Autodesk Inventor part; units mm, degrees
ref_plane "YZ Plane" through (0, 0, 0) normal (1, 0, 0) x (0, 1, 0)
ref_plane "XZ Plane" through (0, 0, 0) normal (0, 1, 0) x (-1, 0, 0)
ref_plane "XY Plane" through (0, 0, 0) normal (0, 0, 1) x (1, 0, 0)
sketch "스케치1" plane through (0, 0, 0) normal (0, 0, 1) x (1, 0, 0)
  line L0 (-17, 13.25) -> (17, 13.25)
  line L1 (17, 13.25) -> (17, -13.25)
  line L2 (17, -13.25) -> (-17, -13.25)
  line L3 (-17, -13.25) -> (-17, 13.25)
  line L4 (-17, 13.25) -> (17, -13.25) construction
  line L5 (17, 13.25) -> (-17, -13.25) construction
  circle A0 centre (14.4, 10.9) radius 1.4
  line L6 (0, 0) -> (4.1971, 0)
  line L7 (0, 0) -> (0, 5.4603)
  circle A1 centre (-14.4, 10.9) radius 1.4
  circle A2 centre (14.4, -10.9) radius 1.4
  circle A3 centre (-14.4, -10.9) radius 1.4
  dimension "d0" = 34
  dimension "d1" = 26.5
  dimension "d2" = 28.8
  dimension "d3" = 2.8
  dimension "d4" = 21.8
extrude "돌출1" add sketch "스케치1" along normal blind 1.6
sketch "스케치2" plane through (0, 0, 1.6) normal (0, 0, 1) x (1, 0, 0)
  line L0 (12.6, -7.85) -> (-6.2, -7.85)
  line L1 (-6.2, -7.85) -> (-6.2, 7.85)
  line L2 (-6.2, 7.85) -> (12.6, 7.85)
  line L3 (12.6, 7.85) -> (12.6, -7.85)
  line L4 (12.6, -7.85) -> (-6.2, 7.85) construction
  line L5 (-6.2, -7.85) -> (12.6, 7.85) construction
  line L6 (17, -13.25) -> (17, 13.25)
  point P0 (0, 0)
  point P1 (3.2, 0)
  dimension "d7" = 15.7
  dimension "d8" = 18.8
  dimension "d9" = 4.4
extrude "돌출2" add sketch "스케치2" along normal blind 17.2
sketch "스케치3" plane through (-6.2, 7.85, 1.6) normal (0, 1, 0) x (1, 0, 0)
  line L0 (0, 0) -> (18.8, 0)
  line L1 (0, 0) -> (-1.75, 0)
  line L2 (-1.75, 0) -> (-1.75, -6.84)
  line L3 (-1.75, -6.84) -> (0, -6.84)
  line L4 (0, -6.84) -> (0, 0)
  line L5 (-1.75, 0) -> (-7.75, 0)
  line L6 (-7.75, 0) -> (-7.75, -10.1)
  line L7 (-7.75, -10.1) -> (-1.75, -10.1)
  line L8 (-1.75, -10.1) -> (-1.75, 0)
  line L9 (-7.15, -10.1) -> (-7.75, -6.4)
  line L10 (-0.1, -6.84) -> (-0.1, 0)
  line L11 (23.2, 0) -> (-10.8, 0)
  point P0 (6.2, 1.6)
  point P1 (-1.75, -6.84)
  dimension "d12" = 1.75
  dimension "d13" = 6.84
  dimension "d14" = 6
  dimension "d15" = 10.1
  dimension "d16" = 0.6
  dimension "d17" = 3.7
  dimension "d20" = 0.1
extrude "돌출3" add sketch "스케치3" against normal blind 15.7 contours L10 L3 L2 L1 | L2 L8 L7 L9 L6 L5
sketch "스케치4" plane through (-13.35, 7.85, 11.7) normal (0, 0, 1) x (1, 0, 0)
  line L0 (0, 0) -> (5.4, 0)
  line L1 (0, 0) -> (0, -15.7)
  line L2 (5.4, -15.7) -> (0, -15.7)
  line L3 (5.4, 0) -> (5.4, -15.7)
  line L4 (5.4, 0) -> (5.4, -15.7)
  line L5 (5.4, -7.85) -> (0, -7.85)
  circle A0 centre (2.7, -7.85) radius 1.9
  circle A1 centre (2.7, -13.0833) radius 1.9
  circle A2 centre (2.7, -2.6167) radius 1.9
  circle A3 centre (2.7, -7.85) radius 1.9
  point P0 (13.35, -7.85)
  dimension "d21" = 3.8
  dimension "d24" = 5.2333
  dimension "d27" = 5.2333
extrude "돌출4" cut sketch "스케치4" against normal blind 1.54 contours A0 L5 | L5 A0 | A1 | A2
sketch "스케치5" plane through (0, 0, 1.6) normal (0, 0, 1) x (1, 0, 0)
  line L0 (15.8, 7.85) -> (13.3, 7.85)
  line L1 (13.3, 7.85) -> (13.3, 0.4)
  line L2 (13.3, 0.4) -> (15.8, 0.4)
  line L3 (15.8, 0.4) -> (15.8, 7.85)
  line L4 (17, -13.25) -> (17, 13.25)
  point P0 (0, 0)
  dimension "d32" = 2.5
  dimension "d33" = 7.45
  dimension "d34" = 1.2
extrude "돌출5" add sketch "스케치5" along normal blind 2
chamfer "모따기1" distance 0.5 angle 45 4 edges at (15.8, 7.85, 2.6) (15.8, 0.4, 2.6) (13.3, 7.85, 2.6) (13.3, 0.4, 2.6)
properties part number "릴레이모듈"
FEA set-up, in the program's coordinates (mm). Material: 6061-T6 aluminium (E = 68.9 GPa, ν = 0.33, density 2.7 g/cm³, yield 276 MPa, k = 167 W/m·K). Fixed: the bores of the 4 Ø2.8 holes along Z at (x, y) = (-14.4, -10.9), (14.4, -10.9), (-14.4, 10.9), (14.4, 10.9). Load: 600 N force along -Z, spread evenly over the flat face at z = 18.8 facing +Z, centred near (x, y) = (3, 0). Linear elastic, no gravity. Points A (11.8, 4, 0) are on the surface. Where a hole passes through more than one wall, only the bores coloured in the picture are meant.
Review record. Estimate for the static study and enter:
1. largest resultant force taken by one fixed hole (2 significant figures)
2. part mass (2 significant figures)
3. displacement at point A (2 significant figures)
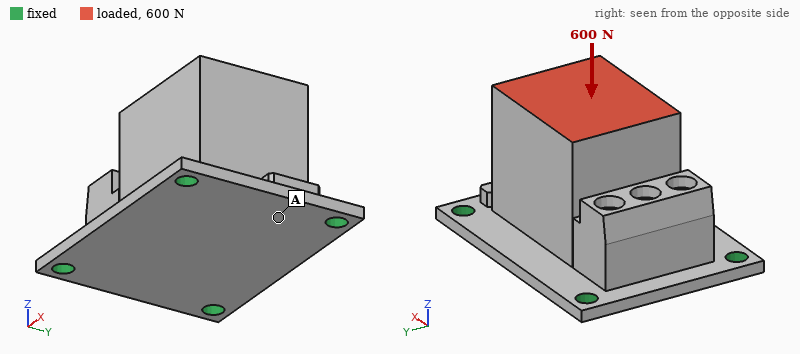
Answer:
210 N
20 g
11 µm
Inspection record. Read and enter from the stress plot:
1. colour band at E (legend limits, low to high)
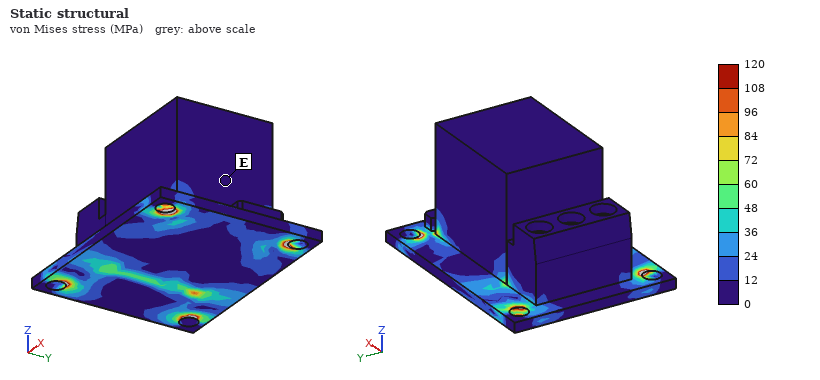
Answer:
0 to 12 MPa
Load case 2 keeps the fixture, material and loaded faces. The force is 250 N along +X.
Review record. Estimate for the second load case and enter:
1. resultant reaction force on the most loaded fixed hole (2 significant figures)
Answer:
130 N
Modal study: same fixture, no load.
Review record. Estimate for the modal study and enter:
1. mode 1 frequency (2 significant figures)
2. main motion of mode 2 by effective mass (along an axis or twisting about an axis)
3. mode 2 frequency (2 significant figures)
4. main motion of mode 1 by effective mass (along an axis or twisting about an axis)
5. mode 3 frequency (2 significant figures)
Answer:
5300 Hz
along Y
7400 Hz
along Z
9500 Hz
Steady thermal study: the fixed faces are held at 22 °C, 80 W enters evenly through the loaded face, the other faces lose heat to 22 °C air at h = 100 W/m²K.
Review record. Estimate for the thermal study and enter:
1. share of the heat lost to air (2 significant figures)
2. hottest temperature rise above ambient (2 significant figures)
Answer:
17 %
73 K
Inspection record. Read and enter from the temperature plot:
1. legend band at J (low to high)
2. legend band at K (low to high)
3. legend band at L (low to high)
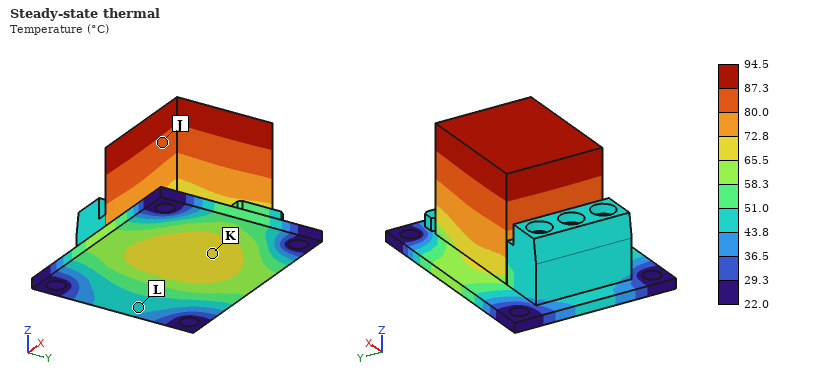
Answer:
80.0 to 87.3 °C
65.5 to 72.8 °C
43.8 to 51.0 °C
